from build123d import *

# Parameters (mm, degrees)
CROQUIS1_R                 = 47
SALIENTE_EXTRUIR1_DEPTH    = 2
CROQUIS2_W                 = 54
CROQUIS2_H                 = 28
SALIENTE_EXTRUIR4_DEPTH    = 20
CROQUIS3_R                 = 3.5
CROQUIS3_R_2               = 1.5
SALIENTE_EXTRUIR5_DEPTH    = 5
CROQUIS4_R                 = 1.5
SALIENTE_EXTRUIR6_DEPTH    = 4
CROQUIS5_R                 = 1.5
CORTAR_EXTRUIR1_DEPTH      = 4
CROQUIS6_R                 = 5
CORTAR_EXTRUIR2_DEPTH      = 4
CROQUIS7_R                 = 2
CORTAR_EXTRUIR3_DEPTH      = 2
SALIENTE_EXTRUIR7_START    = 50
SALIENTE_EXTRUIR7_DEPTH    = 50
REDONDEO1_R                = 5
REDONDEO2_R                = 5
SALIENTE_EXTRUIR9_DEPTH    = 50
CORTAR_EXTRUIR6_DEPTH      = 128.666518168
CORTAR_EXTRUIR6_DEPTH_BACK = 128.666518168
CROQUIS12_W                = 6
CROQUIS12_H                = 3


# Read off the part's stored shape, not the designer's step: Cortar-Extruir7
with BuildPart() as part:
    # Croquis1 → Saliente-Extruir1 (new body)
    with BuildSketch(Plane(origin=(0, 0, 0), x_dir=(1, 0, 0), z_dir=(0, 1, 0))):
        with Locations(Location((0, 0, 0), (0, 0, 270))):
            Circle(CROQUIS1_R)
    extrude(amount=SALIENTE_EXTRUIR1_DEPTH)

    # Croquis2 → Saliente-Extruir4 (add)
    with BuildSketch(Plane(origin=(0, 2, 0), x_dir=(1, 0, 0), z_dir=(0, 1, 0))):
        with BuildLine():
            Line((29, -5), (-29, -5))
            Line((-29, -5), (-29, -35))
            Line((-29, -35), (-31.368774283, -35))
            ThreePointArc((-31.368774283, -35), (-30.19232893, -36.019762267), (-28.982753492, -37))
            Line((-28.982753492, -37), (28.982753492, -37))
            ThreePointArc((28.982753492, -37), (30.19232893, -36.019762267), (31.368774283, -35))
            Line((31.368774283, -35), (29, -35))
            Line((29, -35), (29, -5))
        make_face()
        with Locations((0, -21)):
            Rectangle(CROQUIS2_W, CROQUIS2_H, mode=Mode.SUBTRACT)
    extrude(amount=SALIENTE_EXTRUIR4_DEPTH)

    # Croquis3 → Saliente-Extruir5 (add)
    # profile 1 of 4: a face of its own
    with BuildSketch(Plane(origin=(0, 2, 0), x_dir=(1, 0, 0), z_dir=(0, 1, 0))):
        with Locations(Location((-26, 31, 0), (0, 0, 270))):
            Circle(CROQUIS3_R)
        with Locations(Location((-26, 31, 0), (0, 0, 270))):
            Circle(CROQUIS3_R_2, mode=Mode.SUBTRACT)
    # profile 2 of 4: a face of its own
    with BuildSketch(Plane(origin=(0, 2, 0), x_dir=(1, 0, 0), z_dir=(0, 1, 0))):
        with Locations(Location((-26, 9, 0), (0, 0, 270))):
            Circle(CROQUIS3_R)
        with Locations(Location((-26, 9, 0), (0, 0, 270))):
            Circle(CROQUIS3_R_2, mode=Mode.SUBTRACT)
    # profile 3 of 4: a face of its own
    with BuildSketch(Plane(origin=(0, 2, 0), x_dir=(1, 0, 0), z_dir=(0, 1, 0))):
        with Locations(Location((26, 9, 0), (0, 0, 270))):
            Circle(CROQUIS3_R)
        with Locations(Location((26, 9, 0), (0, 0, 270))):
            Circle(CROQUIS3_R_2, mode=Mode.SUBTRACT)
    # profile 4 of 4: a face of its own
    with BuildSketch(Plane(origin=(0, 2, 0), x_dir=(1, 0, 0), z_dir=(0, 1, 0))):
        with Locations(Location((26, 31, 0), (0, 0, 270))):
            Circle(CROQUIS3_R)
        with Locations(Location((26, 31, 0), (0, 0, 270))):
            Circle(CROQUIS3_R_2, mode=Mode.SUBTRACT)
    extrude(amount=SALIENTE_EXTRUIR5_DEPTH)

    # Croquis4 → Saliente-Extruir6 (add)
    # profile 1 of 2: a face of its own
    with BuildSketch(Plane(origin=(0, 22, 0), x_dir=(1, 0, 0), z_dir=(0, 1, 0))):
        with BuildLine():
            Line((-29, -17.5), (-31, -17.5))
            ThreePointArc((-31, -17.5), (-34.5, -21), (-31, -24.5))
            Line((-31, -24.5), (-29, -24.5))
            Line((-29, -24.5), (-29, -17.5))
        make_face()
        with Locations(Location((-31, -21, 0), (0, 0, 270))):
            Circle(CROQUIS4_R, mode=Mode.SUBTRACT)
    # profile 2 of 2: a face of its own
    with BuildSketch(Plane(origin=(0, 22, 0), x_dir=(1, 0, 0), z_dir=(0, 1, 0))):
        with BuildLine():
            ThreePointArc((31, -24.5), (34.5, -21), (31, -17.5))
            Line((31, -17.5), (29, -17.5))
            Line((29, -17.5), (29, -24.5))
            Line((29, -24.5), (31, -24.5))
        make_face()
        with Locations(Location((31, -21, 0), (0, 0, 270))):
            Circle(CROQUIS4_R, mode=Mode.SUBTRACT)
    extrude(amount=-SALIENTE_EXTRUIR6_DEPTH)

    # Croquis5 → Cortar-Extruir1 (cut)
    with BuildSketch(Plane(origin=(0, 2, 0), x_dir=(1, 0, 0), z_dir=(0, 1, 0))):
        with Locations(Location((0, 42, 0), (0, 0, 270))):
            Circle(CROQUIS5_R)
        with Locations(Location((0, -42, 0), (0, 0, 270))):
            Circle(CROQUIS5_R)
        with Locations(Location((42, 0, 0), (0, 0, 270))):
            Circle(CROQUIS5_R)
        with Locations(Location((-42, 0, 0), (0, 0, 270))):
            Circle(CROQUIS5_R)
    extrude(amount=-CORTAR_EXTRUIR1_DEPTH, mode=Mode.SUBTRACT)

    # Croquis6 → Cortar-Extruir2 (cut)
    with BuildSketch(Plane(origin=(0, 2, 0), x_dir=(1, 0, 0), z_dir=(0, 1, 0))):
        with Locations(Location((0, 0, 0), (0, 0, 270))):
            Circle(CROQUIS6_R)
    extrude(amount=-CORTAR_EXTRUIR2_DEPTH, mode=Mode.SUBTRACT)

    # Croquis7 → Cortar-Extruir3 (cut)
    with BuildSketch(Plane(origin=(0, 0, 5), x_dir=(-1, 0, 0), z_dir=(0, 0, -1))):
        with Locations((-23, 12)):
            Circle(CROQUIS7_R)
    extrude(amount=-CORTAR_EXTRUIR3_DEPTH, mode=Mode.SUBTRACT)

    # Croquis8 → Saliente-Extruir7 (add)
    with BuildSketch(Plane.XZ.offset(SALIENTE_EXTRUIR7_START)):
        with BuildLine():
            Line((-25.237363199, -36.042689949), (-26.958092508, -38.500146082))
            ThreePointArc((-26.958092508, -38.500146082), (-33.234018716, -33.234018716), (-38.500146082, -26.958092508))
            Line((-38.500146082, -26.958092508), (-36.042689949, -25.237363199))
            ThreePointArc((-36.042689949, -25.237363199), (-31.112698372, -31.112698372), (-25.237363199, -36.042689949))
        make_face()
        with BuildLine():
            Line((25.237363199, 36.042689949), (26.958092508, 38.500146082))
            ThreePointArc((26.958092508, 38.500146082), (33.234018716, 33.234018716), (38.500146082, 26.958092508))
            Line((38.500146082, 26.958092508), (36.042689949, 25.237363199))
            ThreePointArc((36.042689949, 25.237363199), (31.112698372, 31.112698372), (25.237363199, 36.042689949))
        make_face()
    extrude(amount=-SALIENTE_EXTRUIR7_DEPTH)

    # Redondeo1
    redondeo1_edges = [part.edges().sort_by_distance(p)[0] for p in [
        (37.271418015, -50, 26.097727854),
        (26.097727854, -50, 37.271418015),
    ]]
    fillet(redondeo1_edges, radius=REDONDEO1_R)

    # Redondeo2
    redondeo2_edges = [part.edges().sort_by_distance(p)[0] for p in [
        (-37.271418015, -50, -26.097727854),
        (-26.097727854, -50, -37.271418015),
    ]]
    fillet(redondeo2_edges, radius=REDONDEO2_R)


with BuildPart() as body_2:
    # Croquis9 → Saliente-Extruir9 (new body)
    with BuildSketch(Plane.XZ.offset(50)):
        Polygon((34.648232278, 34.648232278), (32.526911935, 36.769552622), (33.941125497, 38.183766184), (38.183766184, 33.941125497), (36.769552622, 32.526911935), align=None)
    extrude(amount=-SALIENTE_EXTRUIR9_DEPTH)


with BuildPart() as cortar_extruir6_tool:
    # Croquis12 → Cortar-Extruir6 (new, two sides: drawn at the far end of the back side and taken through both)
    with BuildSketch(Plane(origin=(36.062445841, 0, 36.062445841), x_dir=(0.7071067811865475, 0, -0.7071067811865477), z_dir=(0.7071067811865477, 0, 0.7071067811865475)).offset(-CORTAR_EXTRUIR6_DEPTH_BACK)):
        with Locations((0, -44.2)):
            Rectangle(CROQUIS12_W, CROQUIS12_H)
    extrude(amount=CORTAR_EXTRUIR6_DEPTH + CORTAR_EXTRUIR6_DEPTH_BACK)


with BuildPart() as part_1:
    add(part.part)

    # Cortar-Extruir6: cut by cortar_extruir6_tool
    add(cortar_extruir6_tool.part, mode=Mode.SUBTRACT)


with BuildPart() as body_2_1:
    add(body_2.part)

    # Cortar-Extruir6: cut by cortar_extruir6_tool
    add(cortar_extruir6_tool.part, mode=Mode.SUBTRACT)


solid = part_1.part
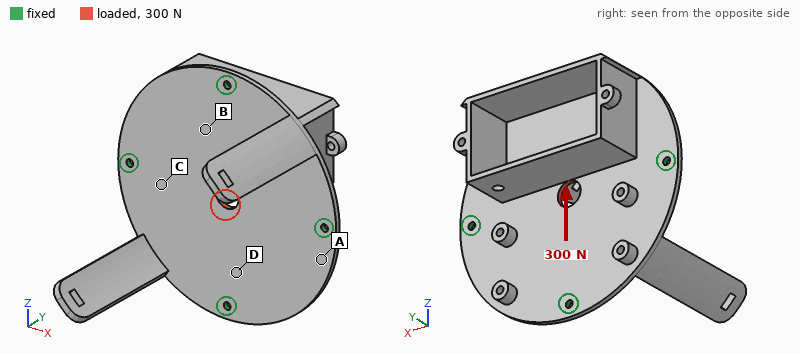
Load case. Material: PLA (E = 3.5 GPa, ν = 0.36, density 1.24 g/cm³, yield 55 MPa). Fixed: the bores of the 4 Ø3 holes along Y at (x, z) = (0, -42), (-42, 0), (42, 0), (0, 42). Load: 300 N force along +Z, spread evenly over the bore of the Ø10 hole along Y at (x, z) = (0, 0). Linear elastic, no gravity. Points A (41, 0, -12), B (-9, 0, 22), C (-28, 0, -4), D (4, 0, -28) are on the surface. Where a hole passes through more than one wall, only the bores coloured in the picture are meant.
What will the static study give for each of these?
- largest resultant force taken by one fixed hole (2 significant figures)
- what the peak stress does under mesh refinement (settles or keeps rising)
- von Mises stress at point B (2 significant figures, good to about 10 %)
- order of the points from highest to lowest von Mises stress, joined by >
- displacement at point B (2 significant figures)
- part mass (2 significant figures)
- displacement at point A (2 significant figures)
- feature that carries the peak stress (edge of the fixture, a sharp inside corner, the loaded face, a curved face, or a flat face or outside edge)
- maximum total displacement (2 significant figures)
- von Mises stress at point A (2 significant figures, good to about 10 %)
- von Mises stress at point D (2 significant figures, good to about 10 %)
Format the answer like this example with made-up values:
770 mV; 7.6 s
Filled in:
96 N; keeps rising; 2.0 MPa; D > B > A > C; 19 µm; 32 g; 6.7 µm; edge of the fixture; 43 µm; 0.98 MPa; 2.7 MPa
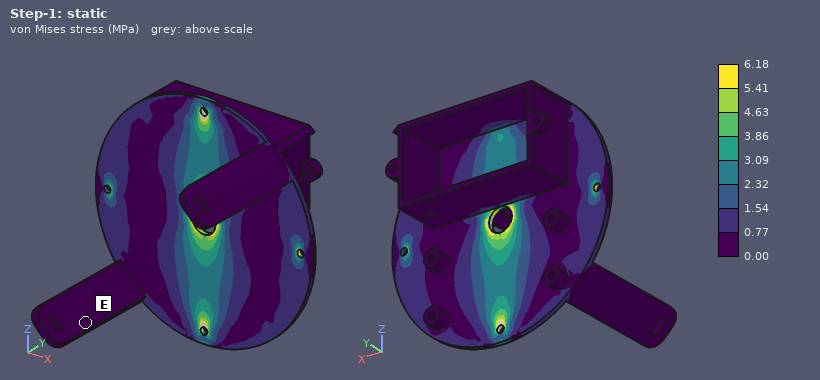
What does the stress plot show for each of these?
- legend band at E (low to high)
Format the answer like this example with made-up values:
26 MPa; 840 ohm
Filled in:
0.00 to 0.77 MPa
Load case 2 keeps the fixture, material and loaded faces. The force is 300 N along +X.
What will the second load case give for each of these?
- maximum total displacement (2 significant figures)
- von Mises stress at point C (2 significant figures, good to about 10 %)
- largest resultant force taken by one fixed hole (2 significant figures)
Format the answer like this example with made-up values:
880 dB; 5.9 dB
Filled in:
37 µm; 2.8 MPa; 95 N
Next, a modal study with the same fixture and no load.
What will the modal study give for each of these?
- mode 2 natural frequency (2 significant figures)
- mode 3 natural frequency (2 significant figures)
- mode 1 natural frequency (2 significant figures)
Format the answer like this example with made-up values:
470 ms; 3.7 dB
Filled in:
270 Hz; 370 Hz; 190 Hz
